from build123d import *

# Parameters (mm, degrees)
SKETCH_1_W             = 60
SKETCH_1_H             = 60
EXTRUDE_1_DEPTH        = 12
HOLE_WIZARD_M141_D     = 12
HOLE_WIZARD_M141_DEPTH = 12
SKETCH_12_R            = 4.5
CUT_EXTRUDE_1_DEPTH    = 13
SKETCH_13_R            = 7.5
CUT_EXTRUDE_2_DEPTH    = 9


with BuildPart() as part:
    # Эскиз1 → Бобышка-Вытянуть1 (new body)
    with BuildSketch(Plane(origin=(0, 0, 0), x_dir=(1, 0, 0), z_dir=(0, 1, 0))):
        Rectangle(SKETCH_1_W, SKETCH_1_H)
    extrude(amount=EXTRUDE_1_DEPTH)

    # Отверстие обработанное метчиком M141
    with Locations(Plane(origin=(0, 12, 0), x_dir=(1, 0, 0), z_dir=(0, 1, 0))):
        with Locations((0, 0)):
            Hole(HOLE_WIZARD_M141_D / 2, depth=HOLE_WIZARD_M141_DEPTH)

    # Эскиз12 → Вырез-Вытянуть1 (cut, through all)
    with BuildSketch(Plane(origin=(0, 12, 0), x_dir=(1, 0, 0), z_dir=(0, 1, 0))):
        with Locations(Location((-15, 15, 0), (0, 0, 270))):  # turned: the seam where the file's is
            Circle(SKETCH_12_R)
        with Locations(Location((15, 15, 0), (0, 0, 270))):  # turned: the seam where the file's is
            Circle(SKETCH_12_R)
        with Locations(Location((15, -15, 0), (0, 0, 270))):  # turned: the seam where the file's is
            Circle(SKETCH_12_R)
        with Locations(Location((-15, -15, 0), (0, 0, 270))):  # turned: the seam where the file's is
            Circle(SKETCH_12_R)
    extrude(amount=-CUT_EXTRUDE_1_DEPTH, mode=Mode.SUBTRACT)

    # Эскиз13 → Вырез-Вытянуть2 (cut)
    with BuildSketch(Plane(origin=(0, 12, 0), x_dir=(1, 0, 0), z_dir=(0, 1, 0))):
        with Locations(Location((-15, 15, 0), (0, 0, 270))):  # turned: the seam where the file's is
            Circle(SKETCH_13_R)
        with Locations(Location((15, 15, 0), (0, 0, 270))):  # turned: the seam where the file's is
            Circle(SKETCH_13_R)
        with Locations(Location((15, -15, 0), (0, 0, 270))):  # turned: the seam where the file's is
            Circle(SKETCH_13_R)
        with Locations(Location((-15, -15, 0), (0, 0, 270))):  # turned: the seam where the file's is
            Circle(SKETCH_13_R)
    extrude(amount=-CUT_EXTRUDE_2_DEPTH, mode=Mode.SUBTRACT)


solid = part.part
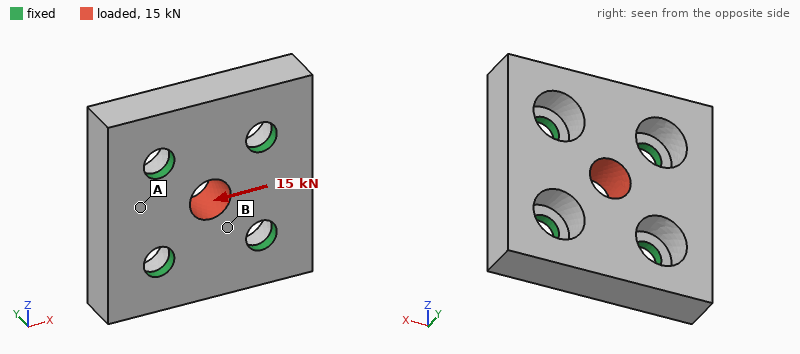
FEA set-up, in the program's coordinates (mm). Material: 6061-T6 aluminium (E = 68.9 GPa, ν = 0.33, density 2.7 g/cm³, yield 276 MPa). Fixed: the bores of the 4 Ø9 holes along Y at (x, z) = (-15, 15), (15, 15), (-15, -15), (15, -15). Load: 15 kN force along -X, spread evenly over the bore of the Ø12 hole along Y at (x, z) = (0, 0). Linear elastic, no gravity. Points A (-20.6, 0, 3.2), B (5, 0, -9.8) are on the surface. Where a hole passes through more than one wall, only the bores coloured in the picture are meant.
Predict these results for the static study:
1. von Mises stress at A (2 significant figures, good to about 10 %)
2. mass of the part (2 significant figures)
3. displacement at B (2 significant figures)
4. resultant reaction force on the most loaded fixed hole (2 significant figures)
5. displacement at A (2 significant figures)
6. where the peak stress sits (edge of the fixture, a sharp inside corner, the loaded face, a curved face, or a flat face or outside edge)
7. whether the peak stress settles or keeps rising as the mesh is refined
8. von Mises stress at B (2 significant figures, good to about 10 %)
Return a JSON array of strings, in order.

["22 MPa", "94 g", "6.2 µm", "4.0 kN", "8.0 µm", "edge of the fixture", "keeps rising", "45 MPa"]
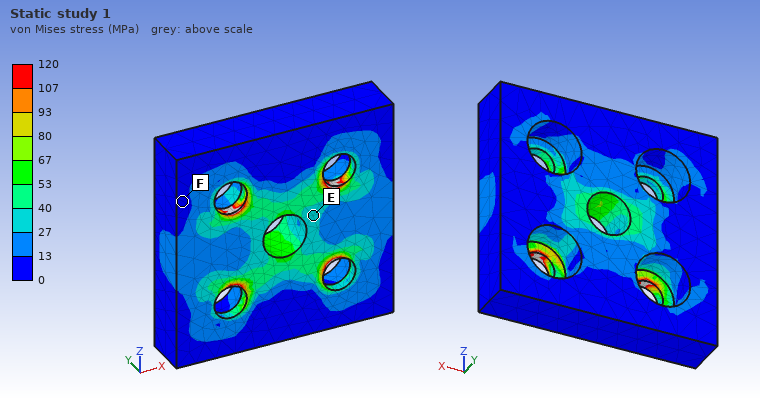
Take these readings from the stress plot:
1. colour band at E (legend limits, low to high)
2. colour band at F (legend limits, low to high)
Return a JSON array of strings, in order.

["27 to 40 MPa", "0 to 13 MPa"]
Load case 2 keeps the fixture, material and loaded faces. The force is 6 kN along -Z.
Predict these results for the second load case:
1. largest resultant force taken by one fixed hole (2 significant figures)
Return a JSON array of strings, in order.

["1.6 kN"]
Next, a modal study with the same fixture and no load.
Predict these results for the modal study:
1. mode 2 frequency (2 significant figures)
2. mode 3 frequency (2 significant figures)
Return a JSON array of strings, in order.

["15 kHz", "17 kHz"]
